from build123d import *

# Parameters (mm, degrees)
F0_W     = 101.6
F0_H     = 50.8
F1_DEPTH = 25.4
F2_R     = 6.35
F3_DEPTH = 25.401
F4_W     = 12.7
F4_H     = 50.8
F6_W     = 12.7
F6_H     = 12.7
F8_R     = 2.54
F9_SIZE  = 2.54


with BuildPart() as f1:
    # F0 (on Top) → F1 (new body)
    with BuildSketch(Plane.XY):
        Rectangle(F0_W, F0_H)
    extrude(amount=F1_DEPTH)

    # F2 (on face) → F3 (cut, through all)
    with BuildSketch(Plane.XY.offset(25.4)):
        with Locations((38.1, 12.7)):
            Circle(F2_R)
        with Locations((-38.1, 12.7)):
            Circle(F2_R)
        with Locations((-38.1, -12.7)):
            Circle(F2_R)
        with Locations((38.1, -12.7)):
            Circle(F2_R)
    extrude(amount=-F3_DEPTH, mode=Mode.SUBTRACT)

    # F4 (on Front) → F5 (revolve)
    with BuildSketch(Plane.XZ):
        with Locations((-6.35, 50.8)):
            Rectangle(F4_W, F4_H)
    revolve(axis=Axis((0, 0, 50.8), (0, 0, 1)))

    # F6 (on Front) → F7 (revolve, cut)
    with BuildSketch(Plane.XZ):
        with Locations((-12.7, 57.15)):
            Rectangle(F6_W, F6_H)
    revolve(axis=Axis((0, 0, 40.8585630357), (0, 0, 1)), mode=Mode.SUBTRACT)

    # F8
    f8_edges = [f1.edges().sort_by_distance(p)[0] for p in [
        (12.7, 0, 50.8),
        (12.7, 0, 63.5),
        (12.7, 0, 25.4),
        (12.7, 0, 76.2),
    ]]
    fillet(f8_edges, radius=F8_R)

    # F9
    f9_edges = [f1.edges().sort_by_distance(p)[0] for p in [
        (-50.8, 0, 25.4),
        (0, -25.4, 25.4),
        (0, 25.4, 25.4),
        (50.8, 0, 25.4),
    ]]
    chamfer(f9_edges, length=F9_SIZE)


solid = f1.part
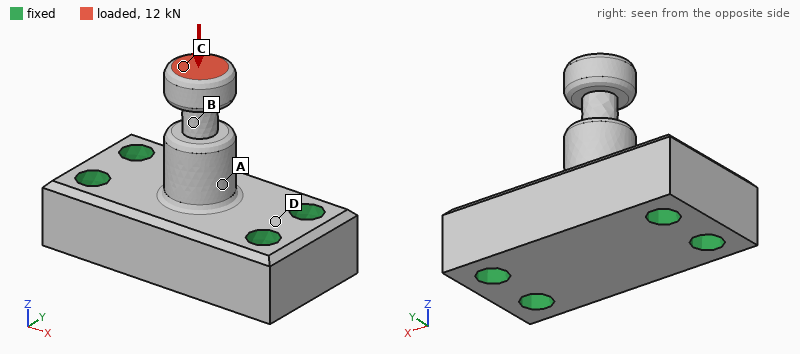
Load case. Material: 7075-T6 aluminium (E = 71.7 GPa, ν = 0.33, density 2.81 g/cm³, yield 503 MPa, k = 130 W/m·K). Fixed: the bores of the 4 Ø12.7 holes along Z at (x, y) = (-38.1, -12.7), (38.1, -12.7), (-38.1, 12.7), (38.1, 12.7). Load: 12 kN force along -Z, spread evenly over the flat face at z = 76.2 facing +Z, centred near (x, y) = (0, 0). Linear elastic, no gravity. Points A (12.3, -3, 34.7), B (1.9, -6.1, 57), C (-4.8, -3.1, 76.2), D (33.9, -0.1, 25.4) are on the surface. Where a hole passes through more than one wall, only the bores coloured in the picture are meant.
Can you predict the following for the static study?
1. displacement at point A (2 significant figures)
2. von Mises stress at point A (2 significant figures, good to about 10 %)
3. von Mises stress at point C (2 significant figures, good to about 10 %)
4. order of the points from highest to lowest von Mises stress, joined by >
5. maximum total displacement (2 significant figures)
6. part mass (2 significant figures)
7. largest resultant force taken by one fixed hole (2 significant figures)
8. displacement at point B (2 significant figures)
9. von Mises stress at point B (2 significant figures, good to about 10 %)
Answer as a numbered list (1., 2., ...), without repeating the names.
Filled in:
1. 12 µm
2. 22 MPa
3. 33 MPa
4. B > C > A > D
5. 46 µm
6. 390 g
7. 3.1 kN
8. 29 µm
9. 93 MPa
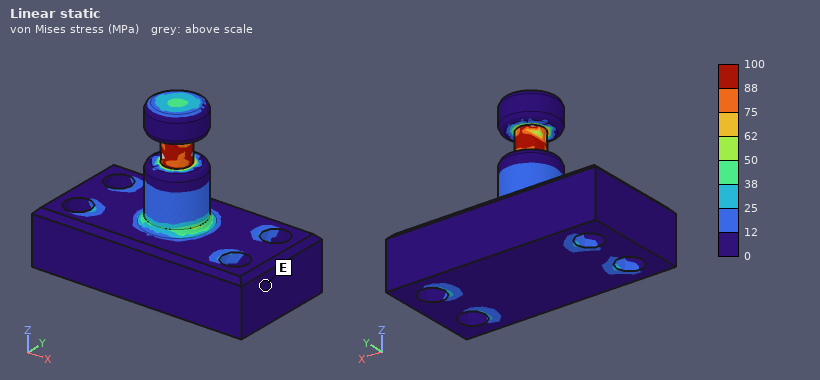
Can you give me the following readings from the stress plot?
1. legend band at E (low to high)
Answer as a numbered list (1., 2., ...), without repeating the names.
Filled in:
1. 0 to 12 MPa
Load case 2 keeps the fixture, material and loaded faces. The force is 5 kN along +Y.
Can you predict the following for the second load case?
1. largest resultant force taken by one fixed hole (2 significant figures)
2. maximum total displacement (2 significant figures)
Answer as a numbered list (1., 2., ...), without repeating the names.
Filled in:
1. 4.2 kN
2. 0.65 mm
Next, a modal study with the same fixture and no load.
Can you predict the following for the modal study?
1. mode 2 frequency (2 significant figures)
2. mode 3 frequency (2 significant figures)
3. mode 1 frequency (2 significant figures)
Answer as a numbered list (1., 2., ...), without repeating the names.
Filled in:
1. 4200 Hz
2. 8400 Hz
3. 4100 Hz
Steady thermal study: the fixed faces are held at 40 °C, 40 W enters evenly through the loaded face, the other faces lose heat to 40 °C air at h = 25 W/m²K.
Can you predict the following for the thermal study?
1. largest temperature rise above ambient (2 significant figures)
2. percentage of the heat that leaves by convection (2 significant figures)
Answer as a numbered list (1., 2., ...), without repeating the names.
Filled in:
1. 66 K
2. 9.4 %
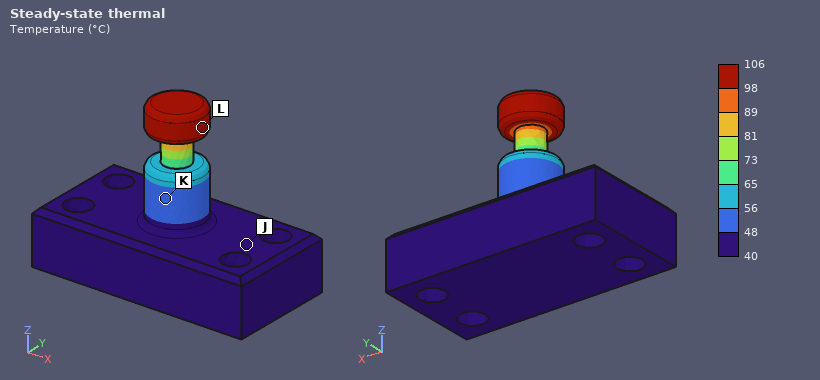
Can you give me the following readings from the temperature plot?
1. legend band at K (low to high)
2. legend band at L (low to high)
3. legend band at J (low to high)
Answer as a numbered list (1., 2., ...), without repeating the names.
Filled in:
1. 48 to 56 °C
2. 98 to 106 °C
3. 40 to 48 °C
